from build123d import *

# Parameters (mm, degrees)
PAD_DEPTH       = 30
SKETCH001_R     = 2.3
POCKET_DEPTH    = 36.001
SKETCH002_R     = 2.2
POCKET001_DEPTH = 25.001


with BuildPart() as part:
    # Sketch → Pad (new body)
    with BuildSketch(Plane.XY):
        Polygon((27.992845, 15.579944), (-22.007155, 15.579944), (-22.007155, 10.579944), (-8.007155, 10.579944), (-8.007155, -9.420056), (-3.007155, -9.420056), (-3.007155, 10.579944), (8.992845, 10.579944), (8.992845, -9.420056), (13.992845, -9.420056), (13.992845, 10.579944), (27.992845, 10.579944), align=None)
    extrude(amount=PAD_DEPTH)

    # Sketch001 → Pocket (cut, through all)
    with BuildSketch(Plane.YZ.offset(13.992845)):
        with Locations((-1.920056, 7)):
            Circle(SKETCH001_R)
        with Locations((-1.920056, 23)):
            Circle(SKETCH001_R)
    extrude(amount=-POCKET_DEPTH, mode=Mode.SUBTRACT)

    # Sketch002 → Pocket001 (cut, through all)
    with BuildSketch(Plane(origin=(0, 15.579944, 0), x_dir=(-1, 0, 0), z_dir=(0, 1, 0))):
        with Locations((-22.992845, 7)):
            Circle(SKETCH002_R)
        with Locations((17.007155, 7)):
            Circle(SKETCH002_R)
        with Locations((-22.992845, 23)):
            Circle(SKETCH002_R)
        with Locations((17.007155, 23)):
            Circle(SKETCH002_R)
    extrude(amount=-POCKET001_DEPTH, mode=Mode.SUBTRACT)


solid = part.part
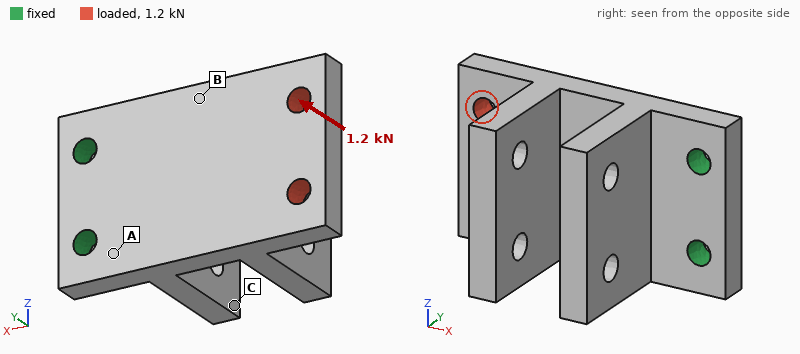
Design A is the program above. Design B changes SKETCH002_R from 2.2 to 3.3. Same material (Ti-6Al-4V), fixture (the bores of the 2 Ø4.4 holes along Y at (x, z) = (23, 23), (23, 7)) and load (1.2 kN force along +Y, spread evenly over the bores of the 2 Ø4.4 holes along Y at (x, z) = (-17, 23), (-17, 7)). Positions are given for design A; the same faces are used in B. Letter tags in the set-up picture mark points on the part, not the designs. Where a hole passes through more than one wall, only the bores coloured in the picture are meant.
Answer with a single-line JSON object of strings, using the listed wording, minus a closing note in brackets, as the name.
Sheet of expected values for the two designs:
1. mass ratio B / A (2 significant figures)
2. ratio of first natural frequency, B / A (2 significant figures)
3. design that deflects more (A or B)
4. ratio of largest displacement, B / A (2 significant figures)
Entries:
{"mass ratio B / A": "0.97", "ratio of first natural frequency, B / A": "1.1", "design that deflects more": "A", "ratio of largest displacement, B / A": "0.90"}
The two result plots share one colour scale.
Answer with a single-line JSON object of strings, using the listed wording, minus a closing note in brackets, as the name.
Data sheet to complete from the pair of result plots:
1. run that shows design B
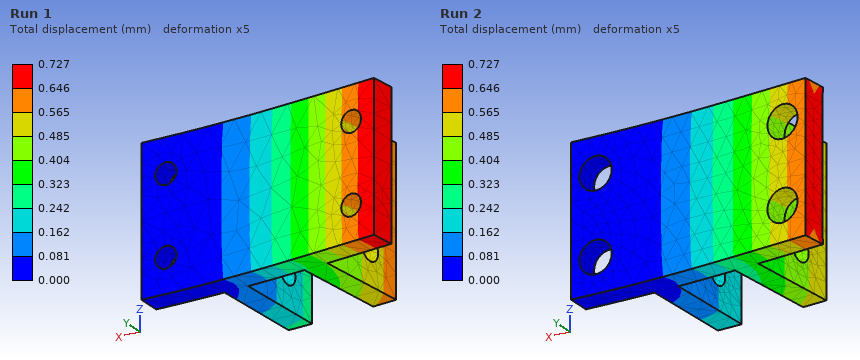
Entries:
{"run that shows design B": "Run 2"}
